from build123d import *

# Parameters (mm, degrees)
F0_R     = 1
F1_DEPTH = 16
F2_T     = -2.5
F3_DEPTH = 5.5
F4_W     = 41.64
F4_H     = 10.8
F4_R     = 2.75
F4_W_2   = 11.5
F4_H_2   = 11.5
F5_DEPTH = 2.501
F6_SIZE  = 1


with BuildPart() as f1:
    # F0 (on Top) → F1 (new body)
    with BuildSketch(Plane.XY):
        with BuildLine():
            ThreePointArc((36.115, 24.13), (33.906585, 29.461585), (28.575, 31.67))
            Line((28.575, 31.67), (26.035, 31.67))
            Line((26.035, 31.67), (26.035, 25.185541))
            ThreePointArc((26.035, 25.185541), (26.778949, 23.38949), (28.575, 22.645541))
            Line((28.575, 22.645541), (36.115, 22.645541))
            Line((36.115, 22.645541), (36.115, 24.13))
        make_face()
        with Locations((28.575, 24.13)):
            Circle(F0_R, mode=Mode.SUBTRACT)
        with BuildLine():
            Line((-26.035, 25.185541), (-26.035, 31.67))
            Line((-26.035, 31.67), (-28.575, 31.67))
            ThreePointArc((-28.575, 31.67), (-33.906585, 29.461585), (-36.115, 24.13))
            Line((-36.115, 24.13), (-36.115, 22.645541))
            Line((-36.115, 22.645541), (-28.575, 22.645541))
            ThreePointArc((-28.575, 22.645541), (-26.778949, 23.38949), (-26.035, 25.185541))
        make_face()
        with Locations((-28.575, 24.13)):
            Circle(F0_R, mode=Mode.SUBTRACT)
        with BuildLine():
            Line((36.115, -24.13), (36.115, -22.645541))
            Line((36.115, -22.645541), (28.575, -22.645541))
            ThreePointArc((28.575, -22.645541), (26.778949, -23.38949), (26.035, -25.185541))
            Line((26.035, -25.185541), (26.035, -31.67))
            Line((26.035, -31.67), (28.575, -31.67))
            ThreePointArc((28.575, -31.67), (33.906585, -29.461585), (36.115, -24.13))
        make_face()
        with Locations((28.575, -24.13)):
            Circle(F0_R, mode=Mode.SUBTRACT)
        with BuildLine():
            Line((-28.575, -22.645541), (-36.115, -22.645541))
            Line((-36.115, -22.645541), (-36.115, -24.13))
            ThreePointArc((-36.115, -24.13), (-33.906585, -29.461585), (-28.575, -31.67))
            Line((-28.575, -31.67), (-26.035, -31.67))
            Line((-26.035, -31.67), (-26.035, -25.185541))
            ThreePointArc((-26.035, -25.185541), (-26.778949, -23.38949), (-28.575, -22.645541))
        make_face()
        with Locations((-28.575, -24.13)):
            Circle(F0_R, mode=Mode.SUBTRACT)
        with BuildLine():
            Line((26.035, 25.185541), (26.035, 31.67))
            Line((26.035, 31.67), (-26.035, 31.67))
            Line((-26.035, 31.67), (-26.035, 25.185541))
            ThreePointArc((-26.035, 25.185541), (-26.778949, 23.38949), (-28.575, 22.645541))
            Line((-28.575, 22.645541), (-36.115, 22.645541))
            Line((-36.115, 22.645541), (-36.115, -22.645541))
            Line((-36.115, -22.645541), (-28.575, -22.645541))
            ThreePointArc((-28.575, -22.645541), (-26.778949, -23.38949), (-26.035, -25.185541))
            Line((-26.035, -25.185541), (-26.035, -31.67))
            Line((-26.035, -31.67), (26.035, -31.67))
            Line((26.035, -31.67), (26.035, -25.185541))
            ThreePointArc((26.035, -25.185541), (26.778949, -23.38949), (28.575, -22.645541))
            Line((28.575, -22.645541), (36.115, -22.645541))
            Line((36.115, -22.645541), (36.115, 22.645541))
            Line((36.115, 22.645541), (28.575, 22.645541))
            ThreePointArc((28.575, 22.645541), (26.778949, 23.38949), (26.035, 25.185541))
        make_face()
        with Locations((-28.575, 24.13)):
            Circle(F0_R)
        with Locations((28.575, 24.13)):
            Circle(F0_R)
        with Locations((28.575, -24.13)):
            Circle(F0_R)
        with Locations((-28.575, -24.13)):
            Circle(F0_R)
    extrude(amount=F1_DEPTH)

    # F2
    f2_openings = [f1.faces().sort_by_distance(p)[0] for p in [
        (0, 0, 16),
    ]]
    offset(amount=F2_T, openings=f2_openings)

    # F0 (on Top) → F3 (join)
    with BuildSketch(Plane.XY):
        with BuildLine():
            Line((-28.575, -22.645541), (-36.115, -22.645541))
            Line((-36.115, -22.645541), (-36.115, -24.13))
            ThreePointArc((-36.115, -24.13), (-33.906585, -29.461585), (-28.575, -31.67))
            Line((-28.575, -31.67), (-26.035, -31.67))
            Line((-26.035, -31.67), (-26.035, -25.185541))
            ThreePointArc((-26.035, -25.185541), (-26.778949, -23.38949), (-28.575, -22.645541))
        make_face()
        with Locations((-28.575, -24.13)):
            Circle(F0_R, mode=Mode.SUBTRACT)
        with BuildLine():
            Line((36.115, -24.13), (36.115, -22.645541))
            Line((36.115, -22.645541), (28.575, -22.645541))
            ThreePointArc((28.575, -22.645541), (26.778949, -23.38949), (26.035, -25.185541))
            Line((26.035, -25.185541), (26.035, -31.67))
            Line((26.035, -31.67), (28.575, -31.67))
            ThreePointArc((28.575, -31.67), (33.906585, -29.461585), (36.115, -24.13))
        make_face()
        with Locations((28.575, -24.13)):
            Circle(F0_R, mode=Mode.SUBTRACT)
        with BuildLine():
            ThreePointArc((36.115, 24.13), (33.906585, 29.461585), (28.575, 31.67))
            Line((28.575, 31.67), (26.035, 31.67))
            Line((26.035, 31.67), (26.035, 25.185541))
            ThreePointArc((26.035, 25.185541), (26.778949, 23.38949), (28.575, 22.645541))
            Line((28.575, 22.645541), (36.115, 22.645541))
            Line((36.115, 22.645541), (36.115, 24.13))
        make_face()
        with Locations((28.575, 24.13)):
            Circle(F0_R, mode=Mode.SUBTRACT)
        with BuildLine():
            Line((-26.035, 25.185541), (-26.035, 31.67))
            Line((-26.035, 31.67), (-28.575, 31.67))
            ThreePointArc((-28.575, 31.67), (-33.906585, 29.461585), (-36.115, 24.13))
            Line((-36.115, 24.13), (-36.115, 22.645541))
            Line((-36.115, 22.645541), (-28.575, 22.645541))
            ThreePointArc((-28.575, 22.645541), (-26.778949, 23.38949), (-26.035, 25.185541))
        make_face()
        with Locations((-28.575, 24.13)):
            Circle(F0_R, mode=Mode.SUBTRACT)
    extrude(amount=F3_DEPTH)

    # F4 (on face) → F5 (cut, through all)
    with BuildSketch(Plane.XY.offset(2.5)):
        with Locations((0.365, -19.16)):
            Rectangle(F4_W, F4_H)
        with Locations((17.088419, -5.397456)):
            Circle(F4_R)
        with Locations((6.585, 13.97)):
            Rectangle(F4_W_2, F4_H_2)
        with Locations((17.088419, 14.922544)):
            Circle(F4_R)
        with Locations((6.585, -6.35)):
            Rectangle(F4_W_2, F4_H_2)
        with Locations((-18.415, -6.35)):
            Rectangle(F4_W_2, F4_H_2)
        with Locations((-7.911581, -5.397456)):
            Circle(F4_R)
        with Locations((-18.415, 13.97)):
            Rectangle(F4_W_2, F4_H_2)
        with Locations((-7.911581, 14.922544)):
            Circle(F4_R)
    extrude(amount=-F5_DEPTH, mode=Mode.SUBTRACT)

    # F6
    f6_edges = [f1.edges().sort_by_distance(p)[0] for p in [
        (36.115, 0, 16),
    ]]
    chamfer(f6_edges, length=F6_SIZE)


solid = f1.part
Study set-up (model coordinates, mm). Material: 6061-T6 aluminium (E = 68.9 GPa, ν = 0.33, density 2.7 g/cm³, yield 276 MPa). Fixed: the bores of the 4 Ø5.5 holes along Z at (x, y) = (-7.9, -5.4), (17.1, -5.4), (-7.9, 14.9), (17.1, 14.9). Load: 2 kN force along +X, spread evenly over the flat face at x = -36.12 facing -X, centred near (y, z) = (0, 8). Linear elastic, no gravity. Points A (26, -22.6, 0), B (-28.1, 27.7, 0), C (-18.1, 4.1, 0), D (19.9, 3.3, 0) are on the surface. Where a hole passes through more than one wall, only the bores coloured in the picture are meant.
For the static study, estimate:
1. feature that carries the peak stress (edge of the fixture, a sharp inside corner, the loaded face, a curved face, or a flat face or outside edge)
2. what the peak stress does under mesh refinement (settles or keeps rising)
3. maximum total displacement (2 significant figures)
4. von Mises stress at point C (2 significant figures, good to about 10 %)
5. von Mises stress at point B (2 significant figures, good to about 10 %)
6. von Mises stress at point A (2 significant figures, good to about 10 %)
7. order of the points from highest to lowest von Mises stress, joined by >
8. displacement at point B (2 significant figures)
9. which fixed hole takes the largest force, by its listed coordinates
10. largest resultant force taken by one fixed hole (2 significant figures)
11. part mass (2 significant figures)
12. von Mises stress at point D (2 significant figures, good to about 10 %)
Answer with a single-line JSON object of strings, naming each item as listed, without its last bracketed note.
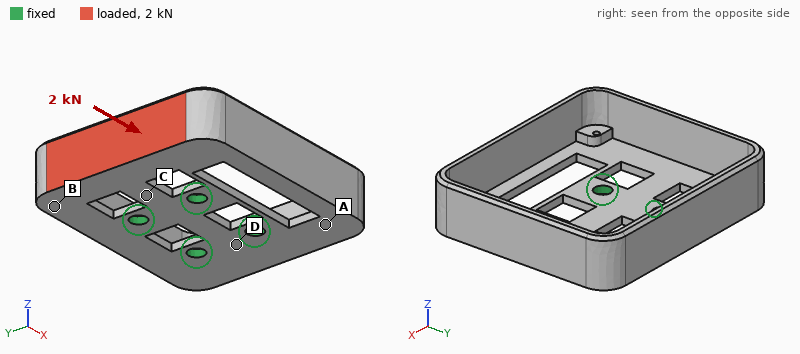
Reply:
{"feature that carries the peak stress": "a sharp inside corner", "what the peak stress does under mesh refinement": "keeps rising", "maximum total displacement": "0.56 mm", "von Mises stress at point C": "49 MPa", "von Mises stress at point B": "63 MPa", "von Mises stress at point A": "15 MPa", "order of the points from highest to lowest von Mises stress, joined by >": "B > C > D > A", "displacement at point B": "0.10 mm", "which fixed hole takes the largest force, by its listed coordinates": "(-7.9, -5.4)", "largest resultant force taken by one fixed hole": "1.0 kN", "part mass": "47 g", "von Mises stress at point D": "34 MPa"}
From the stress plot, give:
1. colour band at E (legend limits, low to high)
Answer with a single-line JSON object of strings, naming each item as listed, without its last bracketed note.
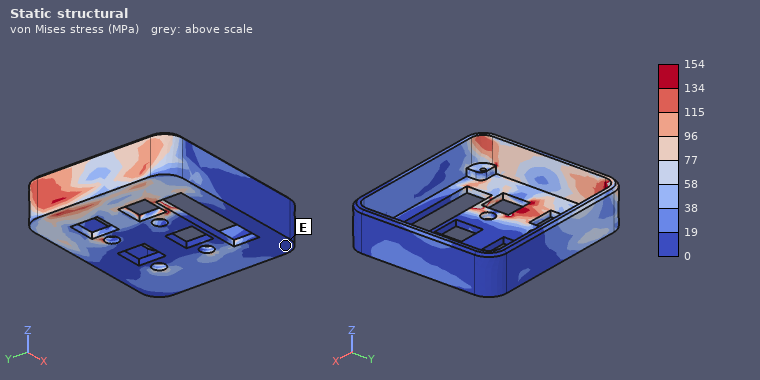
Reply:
{"colour band at E": "0 to 19 MPa"}
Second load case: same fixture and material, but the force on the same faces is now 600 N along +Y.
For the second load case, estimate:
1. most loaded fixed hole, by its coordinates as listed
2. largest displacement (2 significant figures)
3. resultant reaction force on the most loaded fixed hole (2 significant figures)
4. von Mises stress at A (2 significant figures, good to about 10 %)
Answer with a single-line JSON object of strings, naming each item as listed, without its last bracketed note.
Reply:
{"most loaded fixed hole, by its coordinates as listed": "(-7.9, 14.9)", "largest displacement": "0.27 mm", "resultant reaction force on the most loaded fixed hole": "600 N", "von Mises stress at A": "23 MPa"}
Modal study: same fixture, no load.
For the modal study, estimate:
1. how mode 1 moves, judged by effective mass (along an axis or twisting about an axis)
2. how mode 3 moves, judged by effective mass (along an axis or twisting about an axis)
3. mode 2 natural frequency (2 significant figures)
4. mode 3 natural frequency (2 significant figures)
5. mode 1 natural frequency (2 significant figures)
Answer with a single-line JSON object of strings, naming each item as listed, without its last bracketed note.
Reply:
{"how mode 1 moves, judged by effective mass": "along Z", "how mode 3 moves, judged by effective mass": "along Z", "mode 2 natural frequency": "2100 Hz", "mode 3 natural frequency": "2200 Hz", "mode 1 natural frequency": "1100 Hz"}
